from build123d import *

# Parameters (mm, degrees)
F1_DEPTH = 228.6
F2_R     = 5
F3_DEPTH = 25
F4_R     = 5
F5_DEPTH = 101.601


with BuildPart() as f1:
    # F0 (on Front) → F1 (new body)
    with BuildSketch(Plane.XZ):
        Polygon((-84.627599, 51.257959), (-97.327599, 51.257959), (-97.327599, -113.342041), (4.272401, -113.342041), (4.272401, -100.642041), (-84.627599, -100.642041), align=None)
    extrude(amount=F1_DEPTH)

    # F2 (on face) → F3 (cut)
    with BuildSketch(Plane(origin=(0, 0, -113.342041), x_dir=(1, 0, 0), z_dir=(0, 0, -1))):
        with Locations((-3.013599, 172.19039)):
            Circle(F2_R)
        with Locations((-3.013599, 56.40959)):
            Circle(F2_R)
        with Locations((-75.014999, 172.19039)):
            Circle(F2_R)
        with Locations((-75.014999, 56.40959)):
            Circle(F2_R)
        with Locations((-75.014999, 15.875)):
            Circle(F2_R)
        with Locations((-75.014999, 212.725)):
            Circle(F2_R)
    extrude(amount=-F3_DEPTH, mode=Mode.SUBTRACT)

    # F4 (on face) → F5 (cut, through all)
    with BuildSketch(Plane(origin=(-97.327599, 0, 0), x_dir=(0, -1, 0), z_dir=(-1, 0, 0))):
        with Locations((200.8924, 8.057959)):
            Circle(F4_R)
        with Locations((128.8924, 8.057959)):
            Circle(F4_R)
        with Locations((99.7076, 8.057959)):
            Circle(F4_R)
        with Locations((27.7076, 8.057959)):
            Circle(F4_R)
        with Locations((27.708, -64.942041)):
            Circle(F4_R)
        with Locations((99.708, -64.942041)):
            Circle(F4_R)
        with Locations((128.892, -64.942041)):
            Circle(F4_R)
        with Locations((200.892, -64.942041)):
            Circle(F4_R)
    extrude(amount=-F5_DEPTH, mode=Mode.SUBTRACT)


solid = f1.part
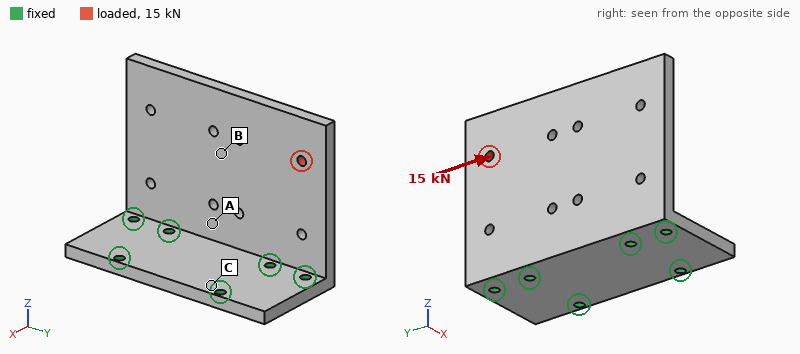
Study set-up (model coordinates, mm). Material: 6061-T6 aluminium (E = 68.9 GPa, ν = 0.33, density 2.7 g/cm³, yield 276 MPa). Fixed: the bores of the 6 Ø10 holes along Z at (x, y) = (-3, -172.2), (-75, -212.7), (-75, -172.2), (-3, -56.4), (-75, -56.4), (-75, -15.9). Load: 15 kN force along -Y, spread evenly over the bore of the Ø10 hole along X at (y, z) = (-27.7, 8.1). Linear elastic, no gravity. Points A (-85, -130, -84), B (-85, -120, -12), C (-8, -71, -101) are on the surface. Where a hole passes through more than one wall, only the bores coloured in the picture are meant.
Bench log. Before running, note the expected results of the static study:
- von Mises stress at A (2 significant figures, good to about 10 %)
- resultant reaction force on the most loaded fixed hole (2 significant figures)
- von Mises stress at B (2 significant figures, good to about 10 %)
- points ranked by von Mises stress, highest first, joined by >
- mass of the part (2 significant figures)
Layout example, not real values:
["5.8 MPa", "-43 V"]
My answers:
["18 MPa", "7.6 kN", "12 MPa", "A > B > C", "1.9 kg"]
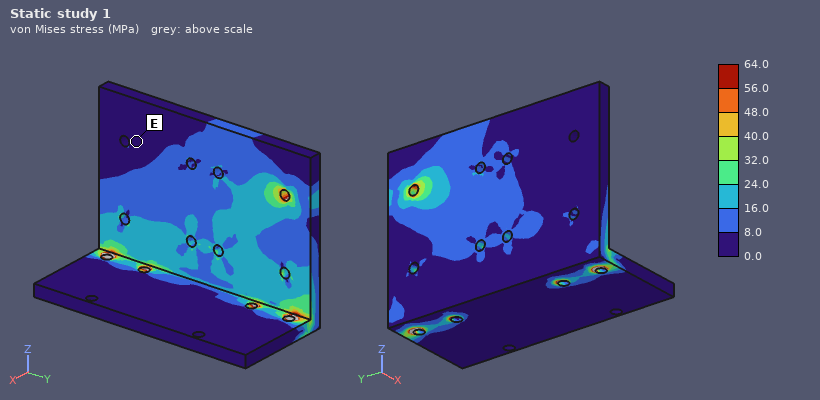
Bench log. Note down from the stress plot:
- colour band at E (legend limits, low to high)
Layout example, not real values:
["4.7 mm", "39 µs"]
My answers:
["0.0 to 8.0 MPa"]
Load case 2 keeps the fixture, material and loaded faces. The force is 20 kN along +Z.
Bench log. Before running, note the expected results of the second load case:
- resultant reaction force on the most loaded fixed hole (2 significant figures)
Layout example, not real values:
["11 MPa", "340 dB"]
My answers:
["11 kN"]
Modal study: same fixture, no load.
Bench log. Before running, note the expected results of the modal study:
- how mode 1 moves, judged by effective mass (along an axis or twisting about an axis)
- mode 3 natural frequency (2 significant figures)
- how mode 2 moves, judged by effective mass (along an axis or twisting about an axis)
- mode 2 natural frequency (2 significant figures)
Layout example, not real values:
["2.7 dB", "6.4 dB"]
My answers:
["along X", "1700 Hz", "twisting about Z", "720 Hz"]
